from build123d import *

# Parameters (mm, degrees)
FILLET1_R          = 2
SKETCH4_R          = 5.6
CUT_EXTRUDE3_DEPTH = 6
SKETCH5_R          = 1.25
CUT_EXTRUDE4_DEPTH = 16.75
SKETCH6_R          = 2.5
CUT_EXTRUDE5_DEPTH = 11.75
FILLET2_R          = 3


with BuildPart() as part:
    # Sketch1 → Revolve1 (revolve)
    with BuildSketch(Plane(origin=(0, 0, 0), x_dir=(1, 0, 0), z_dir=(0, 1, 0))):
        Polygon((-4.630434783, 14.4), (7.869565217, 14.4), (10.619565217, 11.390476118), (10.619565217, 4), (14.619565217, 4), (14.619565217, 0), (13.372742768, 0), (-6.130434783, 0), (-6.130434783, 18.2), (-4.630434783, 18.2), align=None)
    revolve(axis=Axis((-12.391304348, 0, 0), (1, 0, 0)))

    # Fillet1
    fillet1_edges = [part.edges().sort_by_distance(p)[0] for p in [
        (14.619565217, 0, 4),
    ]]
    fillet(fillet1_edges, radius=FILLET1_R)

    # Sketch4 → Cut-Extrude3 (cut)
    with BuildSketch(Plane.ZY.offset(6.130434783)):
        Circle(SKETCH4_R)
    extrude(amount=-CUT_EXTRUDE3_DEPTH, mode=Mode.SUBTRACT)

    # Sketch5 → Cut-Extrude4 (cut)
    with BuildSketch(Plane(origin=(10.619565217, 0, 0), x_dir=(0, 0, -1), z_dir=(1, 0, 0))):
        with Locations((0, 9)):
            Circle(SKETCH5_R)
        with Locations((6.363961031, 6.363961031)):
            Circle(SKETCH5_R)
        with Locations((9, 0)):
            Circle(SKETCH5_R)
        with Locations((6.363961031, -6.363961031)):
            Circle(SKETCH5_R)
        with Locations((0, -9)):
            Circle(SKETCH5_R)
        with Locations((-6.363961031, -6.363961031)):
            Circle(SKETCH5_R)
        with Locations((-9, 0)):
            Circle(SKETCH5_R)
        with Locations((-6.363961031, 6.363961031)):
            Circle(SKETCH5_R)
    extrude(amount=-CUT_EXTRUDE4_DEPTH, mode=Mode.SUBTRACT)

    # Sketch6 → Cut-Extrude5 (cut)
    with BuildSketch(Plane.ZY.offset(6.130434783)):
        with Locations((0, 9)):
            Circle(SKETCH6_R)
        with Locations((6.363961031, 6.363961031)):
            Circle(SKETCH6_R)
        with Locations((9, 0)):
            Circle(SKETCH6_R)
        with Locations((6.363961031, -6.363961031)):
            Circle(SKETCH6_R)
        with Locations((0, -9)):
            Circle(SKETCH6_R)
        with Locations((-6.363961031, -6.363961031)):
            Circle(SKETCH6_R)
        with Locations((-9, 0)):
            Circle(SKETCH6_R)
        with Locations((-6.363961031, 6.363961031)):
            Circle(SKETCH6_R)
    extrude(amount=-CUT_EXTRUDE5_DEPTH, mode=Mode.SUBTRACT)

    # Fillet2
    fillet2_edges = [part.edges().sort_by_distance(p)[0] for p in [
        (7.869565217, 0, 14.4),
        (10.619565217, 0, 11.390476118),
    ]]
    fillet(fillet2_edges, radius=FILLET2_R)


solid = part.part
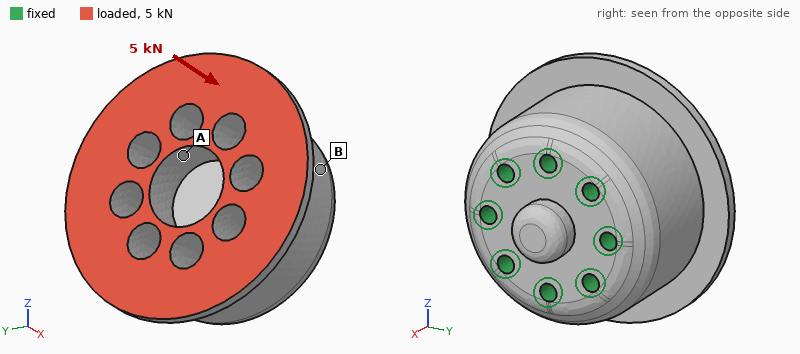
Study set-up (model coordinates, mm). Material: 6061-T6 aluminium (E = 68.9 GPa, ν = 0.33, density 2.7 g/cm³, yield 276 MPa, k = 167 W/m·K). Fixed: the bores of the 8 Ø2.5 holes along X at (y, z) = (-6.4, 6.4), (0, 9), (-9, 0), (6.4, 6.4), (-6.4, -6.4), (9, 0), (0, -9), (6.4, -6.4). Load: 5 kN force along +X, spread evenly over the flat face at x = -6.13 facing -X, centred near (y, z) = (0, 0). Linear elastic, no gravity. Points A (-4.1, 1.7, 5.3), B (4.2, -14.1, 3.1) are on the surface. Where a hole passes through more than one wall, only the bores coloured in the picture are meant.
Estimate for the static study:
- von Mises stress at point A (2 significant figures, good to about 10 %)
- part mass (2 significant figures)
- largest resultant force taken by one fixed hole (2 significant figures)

18 MPa
23 g
630 N
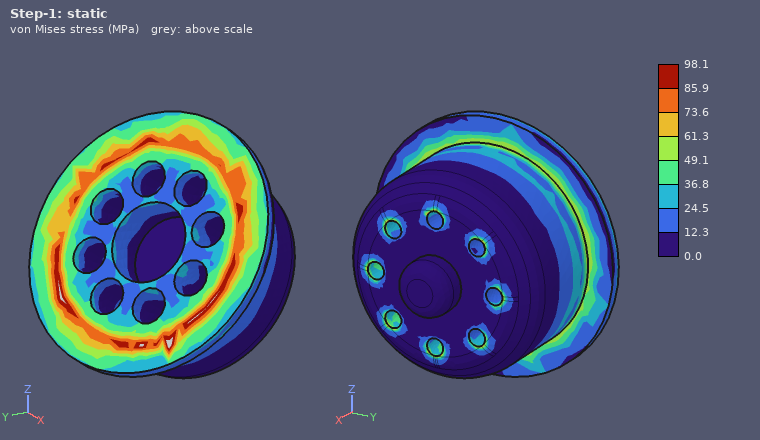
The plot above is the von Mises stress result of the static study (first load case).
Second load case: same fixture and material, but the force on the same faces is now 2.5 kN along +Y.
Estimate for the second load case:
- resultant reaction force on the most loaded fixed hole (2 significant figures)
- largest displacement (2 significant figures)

810 N
18 µm
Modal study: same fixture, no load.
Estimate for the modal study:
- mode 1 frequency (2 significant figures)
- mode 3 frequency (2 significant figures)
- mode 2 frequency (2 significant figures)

29 kHz
38 kHz
29 kHz
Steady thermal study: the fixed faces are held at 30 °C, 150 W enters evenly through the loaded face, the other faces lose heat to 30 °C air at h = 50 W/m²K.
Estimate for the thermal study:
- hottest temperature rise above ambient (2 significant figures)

40 K
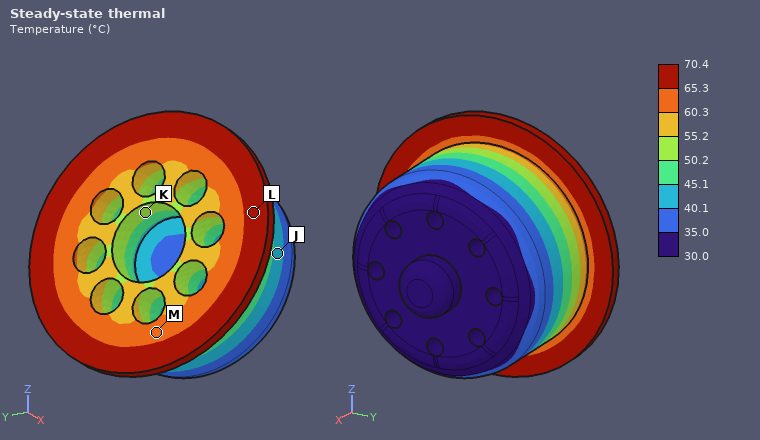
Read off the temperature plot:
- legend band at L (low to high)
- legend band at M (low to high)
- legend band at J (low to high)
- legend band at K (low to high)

65.3 to 70.4 °C
60.3 to 65.3 °C
40.1 to 45.1 °C
50.2 to 55.2 °C
